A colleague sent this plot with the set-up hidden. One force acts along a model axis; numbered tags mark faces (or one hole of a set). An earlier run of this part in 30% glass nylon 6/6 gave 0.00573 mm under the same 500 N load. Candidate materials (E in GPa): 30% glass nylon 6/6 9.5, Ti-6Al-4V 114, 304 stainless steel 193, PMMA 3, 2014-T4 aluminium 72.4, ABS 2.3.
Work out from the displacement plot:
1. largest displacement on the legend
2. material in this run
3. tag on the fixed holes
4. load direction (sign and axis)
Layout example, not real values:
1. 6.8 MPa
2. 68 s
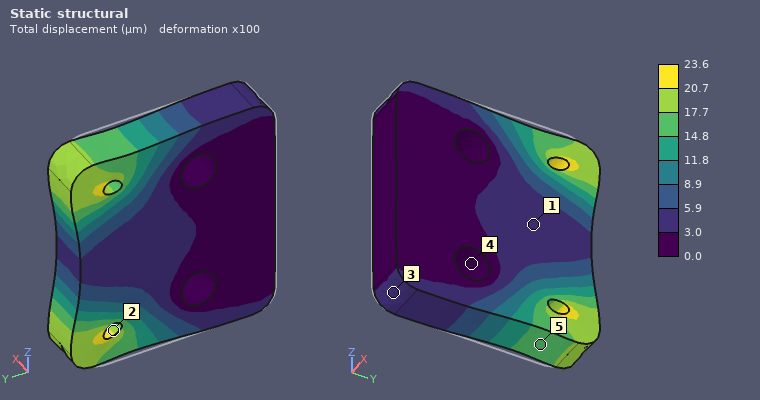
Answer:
1. 23.6 µm
2. ABS
3. 4
4. +Y
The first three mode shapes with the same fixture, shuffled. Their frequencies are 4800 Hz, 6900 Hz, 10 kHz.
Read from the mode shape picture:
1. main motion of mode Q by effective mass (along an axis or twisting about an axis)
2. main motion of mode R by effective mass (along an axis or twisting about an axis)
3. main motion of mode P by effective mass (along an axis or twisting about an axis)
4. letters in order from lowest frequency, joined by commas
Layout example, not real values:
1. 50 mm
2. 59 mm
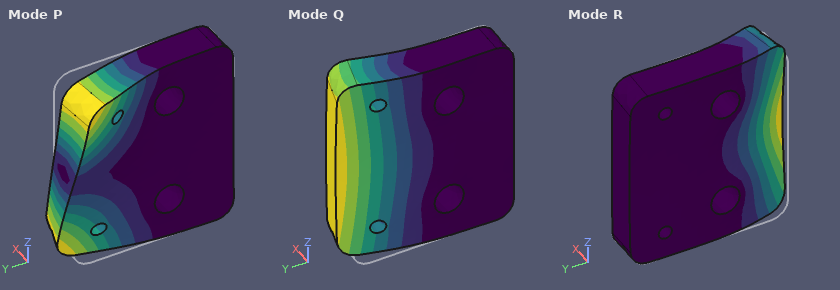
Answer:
1. along X
2. along X
3. twisting about Y
4. Q, P, R
